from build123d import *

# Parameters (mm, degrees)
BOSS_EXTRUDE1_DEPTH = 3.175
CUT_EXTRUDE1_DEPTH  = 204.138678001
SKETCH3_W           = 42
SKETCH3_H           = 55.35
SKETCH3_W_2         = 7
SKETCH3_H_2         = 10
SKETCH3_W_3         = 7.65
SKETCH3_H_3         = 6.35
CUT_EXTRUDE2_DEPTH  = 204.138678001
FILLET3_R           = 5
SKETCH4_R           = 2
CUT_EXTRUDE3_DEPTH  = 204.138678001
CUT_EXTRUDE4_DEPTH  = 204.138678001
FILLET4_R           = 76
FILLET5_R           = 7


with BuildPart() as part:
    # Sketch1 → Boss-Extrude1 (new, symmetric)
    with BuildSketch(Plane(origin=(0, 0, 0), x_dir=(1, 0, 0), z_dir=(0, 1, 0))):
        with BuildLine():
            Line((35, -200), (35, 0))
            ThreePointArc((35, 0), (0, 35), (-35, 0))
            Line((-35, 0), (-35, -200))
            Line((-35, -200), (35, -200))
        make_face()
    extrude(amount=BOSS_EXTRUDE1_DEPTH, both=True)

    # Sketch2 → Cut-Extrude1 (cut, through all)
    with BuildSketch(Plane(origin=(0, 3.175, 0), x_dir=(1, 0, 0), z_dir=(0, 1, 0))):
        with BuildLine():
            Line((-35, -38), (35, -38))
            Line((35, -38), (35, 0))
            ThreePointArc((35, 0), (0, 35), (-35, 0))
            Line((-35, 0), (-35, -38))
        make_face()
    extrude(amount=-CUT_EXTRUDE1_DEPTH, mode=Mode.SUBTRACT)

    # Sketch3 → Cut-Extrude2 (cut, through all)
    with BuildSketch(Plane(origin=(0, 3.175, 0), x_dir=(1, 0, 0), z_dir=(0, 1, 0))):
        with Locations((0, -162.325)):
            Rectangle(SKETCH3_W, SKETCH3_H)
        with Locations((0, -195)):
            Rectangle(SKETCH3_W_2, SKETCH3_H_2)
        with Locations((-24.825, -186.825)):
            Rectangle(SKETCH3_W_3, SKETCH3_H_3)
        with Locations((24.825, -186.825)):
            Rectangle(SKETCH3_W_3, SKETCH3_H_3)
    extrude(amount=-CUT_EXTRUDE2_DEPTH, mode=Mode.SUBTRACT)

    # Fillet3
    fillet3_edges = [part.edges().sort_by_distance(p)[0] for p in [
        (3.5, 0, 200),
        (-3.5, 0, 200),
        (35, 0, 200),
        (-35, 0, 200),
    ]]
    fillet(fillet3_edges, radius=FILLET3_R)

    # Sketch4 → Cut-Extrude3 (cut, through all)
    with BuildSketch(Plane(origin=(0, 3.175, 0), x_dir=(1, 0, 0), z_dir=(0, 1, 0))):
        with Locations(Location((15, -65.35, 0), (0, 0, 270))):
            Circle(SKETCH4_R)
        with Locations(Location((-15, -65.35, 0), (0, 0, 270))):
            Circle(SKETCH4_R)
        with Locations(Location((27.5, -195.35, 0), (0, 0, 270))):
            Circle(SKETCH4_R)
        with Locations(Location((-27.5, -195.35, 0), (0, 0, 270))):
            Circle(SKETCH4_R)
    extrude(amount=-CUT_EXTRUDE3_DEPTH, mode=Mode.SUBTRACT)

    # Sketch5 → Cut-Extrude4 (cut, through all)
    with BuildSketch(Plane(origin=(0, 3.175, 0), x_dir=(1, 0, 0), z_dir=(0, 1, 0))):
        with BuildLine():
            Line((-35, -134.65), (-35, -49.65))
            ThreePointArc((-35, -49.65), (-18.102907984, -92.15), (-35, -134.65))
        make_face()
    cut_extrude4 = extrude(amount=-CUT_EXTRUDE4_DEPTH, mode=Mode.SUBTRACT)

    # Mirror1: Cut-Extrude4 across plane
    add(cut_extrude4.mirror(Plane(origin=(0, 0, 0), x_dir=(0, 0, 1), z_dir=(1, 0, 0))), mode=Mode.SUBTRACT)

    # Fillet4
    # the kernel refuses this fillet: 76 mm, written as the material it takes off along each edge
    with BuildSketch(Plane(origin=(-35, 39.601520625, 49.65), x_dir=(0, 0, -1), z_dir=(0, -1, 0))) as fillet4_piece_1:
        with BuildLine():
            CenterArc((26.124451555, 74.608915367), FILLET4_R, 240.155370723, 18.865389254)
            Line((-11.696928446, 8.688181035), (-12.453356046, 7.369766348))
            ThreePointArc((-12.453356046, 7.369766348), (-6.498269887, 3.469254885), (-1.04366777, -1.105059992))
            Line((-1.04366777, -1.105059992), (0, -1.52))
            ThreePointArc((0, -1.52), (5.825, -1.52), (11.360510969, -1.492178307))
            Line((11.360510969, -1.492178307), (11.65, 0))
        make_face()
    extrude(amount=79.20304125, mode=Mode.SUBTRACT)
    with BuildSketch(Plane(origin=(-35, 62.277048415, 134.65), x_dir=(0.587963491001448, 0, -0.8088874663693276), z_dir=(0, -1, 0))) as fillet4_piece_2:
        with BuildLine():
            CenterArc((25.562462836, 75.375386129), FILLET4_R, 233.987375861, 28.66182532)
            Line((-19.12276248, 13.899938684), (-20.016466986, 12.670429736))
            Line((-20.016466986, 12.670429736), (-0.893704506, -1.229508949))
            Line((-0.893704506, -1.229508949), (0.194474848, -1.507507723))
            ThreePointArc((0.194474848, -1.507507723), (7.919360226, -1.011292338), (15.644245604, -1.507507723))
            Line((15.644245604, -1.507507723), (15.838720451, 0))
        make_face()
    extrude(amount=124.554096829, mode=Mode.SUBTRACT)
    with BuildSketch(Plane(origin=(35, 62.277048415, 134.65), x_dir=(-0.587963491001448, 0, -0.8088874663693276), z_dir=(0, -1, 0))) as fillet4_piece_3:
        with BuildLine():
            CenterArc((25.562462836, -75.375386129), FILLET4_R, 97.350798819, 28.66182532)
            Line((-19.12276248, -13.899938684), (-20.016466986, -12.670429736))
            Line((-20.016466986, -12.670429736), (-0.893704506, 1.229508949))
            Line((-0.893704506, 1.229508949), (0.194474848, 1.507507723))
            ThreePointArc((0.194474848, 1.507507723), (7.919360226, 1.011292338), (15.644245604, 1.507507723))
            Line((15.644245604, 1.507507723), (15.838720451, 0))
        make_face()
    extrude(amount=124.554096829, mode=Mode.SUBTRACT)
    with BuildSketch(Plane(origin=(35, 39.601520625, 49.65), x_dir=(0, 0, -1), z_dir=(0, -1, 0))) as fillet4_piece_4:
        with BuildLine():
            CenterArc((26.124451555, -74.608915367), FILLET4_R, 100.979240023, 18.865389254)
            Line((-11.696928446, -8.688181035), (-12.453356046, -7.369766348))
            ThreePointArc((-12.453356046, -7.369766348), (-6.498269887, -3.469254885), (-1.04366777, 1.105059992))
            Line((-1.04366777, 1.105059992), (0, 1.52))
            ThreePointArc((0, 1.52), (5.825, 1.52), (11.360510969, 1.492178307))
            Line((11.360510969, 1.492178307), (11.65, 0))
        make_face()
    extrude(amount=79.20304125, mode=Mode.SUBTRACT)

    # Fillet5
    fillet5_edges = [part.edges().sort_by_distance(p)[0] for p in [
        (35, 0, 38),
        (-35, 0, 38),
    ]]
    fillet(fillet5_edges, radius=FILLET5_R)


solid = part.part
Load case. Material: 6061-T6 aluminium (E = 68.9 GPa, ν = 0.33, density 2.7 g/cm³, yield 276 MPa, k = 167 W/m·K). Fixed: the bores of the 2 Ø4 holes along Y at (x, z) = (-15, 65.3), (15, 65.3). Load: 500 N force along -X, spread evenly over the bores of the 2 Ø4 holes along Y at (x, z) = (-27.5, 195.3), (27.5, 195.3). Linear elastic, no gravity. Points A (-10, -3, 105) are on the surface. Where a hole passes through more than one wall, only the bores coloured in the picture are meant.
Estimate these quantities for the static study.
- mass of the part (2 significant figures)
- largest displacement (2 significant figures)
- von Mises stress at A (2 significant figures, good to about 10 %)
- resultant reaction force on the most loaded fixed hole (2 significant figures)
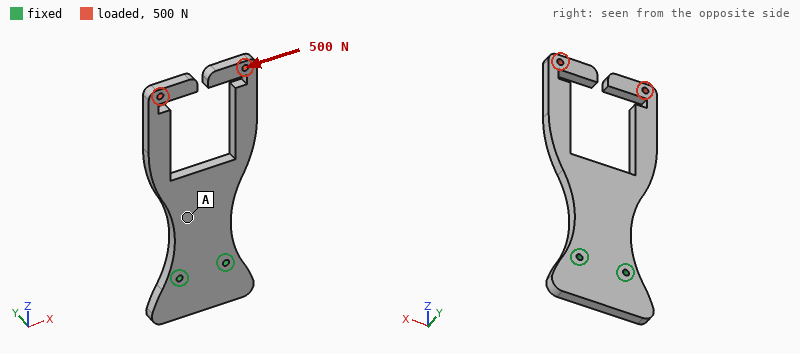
110 g
0.80 mm
13 MPa
2.1 kN
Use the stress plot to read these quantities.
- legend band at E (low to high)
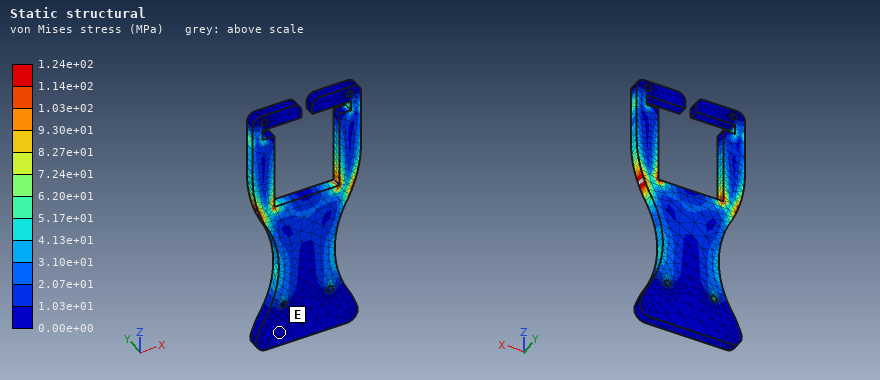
0.00e+00 to 1.03e+01 MPa
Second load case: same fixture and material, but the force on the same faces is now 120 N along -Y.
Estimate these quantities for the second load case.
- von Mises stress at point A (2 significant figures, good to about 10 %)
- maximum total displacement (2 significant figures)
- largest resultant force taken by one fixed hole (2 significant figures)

41 MPa
1.8 mm
60 N
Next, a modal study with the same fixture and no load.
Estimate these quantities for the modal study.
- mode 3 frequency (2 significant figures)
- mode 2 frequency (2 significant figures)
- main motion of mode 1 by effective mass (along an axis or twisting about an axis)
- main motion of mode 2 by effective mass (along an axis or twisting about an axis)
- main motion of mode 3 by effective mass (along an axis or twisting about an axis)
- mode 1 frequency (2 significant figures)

1000 Hz
540 Hz
along Y
twisting about Z
along X
290 Hz
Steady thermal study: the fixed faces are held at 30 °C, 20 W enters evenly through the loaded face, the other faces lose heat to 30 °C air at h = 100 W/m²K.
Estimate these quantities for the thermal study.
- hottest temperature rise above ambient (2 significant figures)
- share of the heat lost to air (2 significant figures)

37 K
83 %
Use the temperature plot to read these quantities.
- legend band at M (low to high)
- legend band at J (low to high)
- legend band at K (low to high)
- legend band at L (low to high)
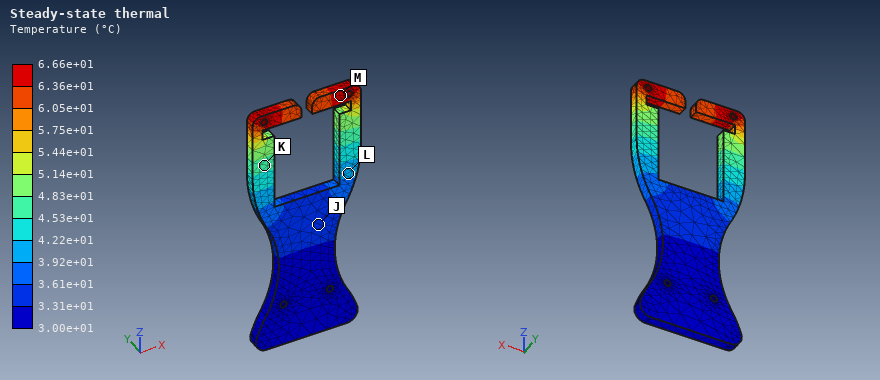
6.36e+01 to 6.66e+01 °C
3.31e+01 to 3.61e+01 °C
4.53e+01 to 4.83e+01 °C
3.92e+01 to 4.22e+01 °C
